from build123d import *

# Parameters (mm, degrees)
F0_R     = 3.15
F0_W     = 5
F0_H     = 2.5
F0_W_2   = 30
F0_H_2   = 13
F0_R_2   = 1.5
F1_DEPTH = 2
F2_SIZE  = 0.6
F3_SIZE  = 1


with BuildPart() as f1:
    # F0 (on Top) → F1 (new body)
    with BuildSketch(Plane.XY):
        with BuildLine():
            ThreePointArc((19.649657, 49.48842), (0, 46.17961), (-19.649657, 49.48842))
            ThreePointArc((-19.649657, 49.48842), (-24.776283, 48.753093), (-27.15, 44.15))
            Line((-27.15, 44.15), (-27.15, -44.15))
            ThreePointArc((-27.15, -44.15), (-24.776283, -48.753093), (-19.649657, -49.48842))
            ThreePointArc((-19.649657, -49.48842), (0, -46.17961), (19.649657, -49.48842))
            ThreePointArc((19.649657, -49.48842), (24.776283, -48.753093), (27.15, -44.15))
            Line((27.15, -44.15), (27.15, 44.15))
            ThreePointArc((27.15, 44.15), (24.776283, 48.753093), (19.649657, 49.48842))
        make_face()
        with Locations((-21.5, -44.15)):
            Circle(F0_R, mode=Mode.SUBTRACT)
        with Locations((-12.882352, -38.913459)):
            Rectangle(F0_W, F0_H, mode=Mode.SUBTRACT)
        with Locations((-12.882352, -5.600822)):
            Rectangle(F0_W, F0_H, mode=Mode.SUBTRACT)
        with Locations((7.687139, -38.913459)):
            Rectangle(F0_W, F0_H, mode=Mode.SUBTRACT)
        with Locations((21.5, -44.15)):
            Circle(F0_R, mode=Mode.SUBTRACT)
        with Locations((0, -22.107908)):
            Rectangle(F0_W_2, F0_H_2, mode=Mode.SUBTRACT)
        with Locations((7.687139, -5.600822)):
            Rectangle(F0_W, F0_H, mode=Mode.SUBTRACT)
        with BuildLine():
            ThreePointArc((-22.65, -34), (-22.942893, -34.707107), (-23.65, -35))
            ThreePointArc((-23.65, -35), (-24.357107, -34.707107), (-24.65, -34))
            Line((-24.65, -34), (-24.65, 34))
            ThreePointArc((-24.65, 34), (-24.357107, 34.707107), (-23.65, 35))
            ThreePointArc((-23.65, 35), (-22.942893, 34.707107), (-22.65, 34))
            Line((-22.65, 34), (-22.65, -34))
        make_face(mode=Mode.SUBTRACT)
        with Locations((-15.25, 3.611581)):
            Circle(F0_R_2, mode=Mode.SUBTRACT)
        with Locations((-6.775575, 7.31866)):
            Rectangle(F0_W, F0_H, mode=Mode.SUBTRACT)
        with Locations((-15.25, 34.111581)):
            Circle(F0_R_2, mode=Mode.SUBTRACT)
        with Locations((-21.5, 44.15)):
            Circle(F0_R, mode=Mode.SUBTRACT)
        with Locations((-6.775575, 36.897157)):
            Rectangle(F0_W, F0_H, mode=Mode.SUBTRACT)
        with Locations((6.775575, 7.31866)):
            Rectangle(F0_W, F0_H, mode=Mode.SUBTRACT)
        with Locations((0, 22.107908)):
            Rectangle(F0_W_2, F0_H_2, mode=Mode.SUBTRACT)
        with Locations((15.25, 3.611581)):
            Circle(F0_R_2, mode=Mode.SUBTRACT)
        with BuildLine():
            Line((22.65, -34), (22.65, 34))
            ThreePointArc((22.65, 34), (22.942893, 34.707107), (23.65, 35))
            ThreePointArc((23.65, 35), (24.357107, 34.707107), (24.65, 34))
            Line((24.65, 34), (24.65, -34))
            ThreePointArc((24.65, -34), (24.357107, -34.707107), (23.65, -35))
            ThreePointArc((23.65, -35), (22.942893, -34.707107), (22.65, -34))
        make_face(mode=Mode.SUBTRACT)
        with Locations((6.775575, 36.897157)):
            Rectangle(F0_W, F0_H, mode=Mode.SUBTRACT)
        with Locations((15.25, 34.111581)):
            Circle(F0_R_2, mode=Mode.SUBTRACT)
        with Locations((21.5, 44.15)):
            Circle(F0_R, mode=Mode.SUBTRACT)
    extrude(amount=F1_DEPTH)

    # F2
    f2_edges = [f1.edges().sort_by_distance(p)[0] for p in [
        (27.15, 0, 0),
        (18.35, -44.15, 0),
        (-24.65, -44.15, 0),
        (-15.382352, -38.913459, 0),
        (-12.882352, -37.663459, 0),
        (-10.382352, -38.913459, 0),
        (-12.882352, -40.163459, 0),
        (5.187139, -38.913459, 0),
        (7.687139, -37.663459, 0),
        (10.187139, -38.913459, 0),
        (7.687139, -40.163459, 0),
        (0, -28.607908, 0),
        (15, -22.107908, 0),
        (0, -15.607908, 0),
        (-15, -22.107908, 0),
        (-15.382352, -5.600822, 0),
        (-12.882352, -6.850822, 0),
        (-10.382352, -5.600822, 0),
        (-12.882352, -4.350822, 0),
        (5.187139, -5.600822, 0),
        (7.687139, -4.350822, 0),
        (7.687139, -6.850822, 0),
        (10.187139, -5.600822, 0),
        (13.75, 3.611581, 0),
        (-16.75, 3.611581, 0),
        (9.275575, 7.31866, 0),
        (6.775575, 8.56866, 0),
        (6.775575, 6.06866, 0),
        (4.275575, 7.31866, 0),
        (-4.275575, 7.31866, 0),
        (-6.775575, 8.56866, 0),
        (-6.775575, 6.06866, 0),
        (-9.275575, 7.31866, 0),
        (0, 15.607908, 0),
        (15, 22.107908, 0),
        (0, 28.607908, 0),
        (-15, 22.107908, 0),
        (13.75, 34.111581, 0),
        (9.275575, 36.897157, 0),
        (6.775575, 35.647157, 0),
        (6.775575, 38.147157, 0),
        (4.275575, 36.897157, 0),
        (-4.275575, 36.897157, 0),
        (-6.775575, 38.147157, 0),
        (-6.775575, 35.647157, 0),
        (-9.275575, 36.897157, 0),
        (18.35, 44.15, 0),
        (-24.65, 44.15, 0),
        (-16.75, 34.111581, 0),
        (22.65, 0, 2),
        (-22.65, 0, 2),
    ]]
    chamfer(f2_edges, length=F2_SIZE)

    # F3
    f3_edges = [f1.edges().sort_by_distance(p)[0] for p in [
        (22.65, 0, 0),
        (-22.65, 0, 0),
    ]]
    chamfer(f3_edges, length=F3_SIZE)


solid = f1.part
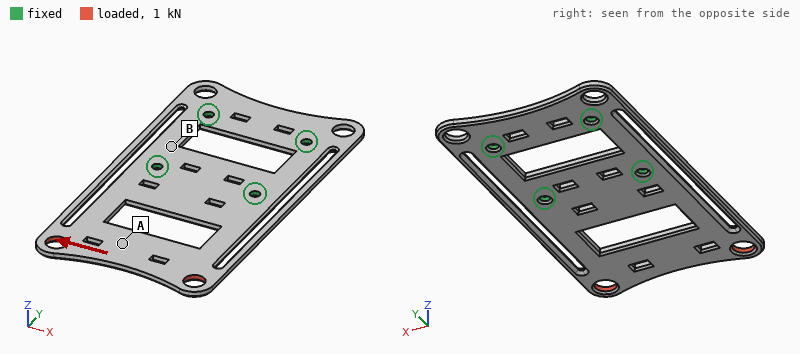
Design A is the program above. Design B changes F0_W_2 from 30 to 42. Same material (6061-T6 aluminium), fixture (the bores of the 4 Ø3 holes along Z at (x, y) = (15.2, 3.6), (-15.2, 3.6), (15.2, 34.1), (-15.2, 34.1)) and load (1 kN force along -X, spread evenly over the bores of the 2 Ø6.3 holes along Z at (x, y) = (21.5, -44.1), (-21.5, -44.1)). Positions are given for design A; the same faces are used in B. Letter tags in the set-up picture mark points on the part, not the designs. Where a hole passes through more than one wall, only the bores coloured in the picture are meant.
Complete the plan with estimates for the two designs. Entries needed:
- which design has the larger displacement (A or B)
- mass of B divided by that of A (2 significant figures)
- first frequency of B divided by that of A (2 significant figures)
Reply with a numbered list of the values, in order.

1. B
2. 0.91
3. 0.67
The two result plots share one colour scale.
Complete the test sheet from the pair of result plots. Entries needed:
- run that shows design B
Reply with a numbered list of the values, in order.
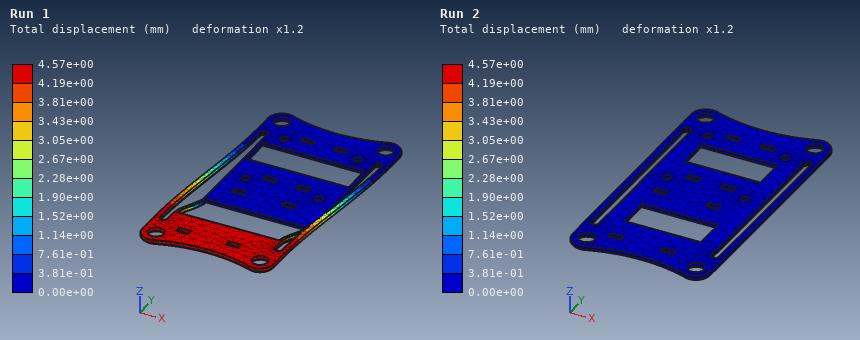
1. Run 1
